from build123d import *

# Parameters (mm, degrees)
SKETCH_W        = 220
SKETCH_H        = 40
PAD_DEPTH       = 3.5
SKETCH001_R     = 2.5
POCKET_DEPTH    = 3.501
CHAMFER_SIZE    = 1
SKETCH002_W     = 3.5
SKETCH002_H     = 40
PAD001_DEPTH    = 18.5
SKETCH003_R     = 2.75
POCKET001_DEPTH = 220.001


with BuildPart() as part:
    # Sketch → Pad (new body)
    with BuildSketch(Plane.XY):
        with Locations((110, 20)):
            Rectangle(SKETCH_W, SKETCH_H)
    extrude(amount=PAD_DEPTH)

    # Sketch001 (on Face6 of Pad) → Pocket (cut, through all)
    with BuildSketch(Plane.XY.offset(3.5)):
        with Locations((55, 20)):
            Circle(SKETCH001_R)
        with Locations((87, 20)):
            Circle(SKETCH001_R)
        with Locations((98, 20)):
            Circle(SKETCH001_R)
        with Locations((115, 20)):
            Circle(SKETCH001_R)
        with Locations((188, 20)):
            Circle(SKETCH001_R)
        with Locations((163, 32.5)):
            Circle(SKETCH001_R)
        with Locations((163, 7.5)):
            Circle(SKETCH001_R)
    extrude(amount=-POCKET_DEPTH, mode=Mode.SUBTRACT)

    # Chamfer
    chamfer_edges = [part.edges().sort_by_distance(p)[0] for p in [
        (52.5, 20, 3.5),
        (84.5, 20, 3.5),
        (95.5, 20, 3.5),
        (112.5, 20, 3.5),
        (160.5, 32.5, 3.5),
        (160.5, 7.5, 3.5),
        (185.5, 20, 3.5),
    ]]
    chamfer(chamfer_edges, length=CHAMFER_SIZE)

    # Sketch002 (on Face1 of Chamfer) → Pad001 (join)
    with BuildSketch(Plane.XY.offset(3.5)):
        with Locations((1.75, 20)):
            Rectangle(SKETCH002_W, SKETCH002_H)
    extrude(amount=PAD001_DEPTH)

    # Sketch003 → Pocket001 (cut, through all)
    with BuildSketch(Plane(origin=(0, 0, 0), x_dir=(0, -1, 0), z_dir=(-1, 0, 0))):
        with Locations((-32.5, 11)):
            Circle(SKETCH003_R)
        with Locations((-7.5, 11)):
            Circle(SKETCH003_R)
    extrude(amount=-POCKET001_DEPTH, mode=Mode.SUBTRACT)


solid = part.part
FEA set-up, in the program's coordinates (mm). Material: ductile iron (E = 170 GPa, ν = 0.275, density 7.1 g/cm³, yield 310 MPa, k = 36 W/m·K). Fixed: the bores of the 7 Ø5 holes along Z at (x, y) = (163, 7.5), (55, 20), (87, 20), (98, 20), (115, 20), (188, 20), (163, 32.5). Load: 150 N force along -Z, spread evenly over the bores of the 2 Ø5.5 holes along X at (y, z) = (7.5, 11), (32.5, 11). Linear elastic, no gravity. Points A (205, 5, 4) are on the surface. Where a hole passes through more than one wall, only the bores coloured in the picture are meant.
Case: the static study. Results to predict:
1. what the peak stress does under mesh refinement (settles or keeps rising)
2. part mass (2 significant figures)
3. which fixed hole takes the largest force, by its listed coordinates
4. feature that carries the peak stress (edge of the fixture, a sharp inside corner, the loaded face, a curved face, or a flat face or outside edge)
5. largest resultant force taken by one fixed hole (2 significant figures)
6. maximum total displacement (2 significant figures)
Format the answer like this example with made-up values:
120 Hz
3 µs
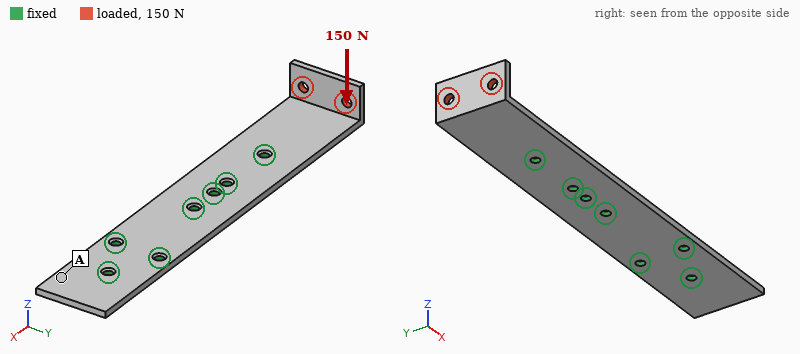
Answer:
keeps rising
230 g
(55, 20)
edge of the fixture
290 N
0.40 mm
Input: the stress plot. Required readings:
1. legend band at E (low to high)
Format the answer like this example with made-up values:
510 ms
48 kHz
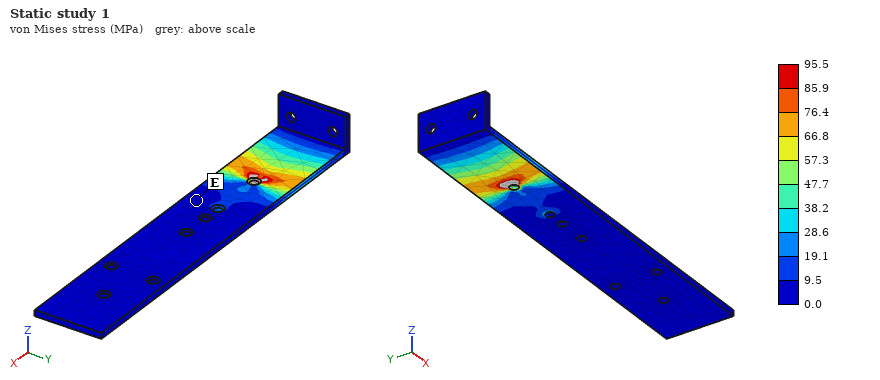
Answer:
0.0 to 9.5 MPa
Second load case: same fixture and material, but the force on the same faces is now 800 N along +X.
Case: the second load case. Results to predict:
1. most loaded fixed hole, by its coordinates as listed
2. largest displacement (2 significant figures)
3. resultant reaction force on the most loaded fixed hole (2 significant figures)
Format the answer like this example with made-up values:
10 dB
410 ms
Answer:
(55, 20)
0.60 mm
470 N
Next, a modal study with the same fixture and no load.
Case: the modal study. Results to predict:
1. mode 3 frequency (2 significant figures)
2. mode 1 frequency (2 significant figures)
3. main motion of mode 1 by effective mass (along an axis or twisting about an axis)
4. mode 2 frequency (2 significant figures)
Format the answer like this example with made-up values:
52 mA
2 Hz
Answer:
2400 Hz
570 Hz
along Z
1500 Hz
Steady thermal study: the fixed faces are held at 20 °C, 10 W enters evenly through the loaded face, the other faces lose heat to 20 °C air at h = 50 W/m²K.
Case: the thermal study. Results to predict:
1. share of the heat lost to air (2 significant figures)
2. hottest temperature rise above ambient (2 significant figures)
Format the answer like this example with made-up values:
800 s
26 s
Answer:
81 %
54 K
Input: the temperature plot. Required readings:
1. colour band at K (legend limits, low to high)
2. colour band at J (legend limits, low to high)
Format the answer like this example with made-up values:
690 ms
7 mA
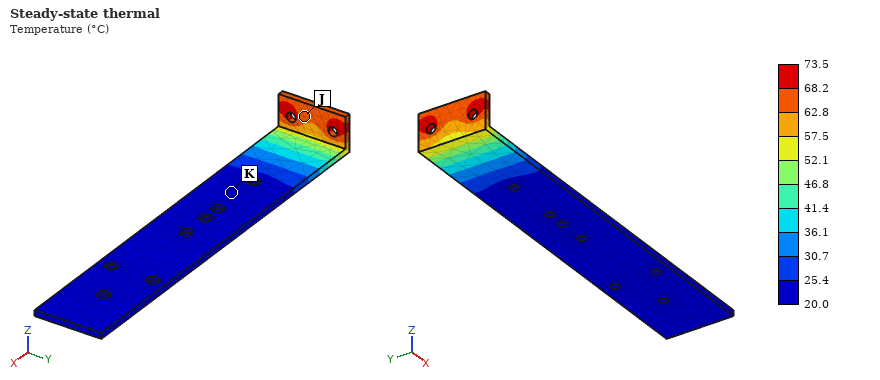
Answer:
20.0 to 25.4 °C
62.8 to 68.2 °C
